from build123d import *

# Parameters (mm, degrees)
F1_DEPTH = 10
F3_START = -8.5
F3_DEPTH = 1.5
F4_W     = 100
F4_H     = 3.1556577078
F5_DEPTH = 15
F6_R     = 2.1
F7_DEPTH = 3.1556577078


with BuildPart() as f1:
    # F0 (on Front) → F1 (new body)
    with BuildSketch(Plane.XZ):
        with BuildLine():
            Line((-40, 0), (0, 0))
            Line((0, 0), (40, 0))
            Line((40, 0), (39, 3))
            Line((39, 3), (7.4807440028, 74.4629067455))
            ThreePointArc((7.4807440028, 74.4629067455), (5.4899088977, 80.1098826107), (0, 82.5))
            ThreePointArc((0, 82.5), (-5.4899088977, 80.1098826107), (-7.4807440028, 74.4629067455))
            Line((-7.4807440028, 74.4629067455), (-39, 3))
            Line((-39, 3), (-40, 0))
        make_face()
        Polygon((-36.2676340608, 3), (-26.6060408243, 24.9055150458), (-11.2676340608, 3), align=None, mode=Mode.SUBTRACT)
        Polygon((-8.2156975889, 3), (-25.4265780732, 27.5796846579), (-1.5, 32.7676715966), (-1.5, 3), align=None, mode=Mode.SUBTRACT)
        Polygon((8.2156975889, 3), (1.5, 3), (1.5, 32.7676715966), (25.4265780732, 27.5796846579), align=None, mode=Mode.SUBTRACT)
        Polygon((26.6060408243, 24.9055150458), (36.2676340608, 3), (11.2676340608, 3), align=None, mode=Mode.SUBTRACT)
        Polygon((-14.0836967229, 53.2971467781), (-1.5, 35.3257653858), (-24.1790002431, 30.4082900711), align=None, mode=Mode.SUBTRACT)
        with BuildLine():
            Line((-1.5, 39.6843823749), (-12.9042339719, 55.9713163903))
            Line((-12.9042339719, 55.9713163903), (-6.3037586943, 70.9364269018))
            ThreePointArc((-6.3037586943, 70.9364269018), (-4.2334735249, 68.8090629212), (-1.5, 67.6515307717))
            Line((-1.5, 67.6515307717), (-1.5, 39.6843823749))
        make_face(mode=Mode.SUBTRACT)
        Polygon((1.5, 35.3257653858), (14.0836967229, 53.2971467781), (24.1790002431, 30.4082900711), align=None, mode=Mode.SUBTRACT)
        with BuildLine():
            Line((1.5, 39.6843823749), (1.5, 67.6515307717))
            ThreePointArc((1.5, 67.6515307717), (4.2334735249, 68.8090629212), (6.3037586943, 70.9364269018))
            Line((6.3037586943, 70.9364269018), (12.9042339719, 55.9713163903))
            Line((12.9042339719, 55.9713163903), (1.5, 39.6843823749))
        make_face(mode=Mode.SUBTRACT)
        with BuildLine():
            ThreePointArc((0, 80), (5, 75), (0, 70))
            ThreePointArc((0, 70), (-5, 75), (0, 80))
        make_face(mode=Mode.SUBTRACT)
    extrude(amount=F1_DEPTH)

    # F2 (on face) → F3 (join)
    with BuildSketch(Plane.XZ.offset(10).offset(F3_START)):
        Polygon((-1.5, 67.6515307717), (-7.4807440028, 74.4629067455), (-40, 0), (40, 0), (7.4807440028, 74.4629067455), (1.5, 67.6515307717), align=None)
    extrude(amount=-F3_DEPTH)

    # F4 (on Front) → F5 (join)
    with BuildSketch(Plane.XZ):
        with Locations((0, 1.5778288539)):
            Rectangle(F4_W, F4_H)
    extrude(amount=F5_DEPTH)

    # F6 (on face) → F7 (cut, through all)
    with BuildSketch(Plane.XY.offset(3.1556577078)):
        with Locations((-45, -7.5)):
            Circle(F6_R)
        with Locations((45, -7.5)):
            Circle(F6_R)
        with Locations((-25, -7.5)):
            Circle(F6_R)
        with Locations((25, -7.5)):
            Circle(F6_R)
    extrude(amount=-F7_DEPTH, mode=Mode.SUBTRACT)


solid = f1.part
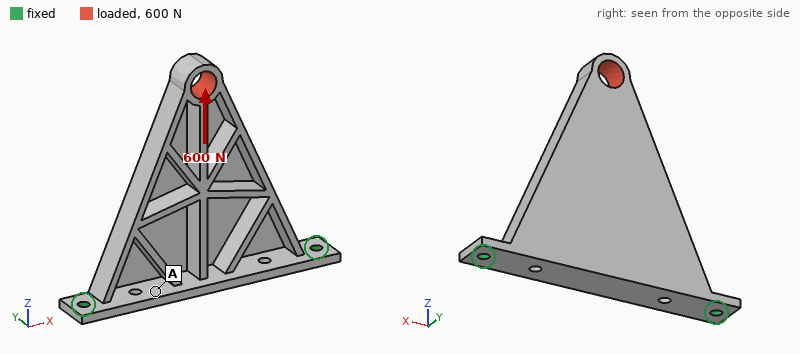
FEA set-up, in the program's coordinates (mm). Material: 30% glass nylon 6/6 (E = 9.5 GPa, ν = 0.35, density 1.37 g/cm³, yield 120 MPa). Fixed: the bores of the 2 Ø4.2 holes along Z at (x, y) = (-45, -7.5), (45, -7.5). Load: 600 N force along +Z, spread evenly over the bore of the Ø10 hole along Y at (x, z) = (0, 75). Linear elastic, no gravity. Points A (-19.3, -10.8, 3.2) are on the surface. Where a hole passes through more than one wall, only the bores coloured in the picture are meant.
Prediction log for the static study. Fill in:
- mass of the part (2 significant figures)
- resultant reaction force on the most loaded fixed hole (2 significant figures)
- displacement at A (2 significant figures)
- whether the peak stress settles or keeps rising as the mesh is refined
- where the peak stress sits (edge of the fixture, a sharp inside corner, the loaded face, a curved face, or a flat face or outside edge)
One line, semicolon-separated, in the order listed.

25 g; 340 N; 0.079 mm; keeps rising; edge of the fixture
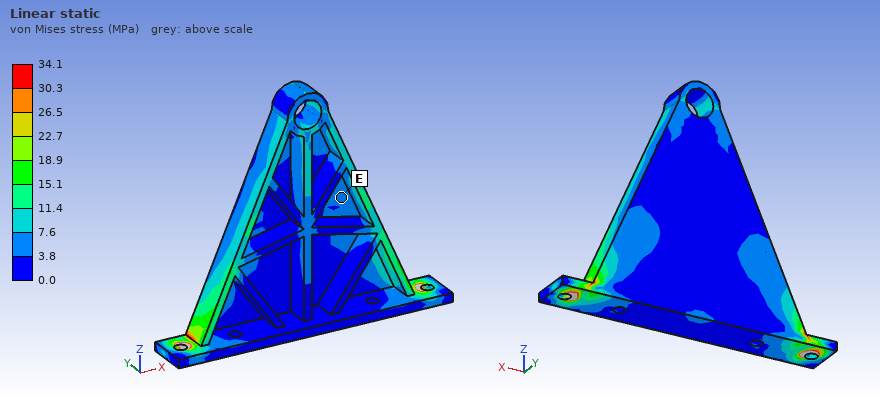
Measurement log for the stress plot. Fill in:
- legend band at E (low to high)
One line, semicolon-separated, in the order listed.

3.8 to 7.6 MPa
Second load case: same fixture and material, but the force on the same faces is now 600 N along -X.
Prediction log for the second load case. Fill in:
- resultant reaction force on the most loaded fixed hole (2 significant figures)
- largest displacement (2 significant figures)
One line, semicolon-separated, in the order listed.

620 N; 0.70 mm
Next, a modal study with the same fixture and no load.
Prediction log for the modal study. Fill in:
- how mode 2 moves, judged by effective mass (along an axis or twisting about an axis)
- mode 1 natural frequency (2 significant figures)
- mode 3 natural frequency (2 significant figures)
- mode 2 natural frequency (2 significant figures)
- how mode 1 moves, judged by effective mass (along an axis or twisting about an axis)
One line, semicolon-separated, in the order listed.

along X; 320 Hz; 2200 Hz; 2000 Hz; along Y
